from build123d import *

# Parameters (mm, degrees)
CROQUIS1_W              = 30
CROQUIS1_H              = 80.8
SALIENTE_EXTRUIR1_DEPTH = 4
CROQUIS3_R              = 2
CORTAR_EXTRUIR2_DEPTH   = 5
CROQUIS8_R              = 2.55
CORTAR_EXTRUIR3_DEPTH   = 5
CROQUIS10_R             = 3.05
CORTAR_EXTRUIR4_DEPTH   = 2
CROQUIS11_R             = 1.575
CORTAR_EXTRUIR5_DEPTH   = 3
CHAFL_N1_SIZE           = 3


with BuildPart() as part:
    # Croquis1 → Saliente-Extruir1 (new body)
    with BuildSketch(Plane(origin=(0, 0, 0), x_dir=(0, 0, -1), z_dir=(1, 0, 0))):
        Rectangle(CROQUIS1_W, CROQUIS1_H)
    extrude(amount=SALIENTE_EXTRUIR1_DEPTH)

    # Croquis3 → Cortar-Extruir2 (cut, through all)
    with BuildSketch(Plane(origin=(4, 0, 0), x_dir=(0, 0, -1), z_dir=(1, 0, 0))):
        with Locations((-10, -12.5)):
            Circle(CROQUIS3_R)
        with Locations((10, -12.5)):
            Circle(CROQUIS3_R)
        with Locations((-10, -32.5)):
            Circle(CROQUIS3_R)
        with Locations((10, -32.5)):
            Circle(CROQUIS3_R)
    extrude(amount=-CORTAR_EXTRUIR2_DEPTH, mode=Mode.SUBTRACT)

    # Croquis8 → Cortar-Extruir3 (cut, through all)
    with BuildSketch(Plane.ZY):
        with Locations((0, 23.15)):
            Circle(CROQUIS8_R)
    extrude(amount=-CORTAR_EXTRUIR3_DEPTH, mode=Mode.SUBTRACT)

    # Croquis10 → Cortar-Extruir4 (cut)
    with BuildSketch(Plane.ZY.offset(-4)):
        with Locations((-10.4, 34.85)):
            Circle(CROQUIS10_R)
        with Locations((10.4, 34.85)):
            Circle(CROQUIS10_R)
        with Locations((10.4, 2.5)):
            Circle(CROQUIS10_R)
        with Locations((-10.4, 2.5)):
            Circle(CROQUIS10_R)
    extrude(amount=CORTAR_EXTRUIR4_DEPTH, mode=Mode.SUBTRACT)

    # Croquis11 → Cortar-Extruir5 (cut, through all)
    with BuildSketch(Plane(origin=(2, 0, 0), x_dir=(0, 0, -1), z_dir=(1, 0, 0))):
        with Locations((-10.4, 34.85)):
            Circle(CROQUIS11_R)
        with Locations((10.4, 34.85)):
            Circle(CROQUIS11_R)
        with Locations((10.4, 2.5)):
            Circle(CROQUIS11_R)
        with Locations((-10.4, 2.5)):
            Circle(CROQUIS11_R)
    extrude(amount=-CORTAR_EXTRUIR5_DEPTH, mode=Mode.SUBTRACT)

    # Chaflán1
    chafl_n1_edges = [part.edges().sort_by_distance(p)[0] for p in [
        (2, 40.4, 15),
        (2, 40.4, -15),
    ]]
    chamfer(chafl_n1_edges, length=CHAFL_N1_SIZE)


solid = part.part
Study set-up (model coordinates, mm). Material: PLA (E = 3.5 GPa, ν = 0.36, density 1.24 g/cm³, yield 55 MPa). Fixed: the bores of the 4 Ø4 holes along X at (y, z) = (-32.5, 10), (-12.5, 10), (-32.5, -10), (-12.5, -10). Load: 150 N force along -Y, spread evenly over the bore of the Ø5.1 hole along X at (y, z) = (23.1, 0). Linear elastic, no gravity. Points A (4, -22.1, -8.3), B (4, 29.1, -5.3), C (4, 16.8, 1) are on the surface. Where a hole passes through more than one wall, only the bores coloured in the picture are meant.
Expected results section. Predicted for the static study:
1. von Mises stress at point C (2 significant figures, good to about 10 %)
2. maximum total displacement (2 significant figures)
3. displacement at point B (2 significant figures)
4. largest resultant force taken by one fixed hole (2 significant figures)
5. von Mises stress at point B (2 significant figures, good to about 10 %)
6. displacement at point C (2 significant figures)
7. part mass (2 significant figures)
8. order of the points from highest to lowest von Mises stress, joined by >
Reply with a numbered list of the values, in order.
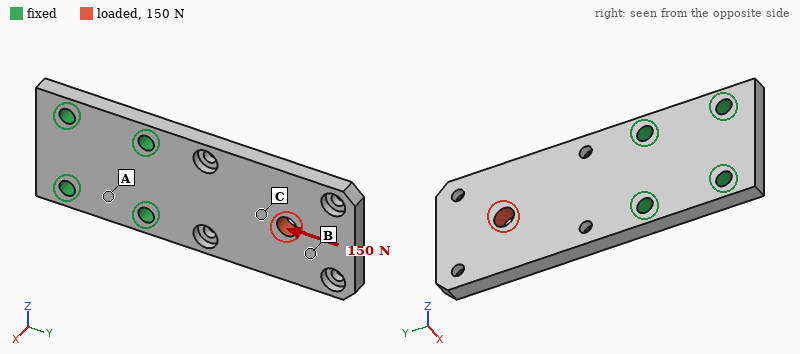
1. 2.2 MPa
2. 29 µm
3. 23 µm
4. 68 N
5. 0.92 MPa
6. 17 µm
7. 11 g
8. C > B > A
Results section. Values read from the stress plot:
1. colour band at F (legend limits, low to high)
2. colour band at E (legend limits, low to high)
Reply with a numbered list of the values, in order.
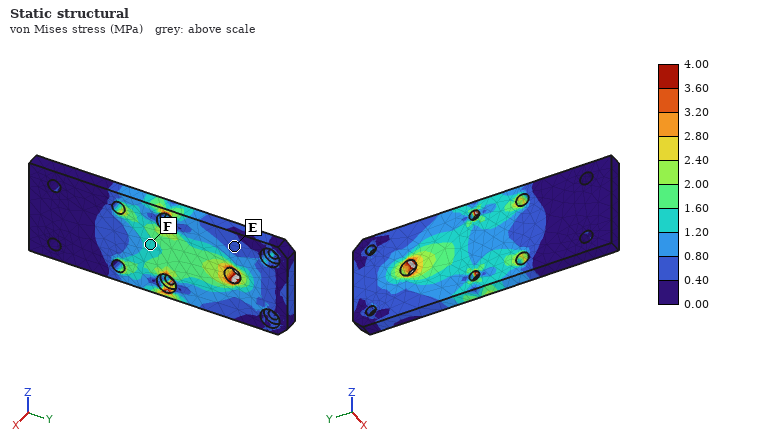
1. 1.20 to 1.60 MPa
2. 0.40 to 0.80 MPa
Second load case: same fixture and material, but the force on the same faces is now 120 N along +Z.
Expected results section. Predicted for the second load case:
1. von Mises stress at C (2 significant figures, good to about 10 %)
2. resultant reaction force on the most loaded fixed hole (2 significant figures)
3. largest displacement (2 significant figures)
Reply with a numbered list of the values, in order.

1. 2.6 MPa
2. 190 N
3. 0.16 mm
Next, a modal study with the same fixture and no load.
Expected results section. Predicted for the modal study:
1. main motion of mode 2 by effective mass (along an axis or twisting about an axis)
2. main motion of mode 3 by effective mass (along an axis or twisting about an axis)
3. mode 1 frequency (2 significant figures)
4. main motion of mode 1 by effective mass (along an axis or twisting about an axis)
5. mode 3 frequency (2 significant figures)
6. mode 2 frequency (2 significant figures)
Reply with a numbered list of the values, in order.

1. twisting about Y
2. along Z
3. 400 Hz
4. along X
5. 2300 Hz
6. 1500 Hz
